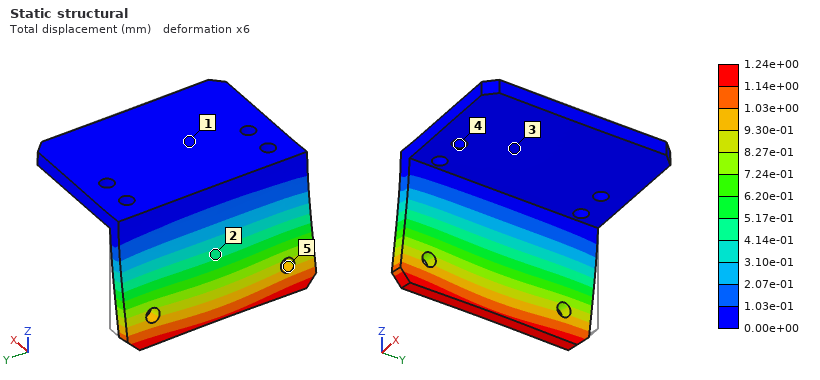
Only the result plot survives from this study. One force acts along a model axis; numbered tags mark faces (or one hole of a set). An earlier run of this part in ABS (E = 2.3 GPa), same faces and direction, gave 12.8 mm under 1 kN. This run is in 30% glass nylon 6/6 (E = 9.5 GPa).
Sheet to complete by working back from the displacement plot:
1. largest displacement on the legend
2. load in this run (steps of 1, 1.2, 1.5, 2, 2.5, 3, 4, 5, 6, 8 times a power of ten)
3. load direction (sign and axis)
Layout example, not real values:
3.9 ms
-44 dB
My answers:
1.24e+00 mm
400 N
-X
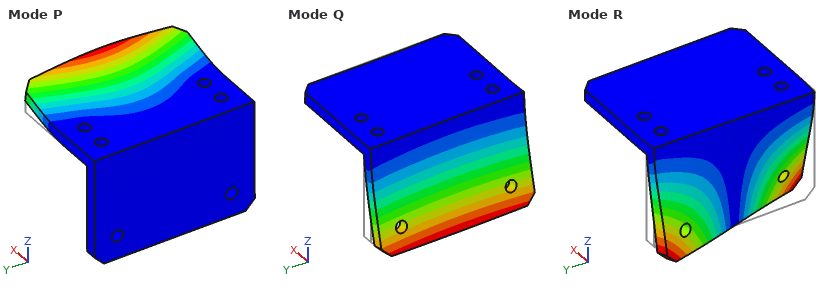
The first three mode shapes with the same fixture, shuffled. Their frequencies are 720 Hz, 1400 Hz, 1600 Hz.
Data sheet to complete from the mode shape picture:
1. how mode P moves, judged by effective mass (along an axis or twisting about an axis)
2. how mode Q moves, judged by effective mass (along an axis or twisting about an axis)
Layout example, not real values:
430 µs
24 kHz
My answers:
along Z
along X
